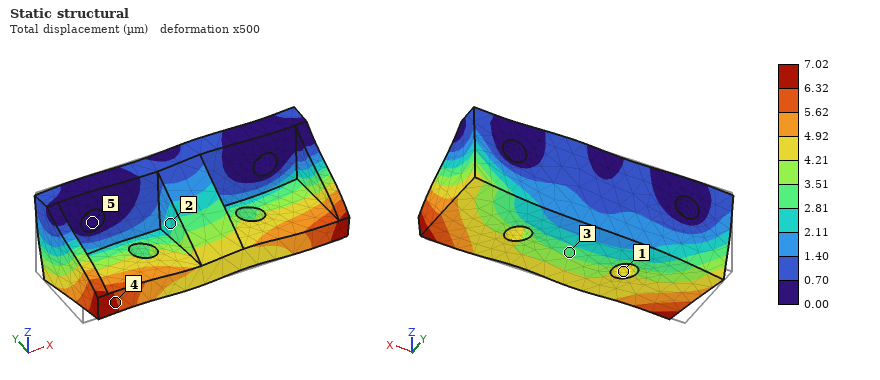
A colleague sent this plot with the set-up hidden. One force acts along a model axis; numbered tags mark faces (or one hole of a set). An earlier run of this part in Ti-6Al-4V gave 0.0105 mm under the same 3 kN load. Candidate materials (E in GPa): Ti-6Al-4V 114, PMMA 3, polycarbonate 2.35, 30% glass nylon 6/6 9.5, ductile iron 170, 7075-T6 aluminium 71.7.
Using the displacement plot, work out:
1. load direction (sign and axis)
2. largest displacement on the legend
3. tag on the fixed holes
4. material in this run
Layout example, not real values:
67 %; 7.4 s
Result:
+X; 7.02 µm; 5; ductile iron
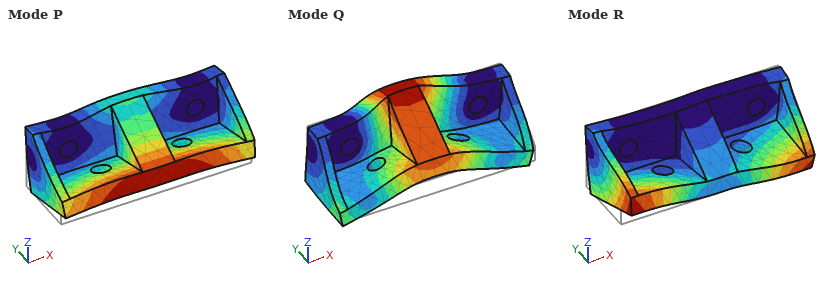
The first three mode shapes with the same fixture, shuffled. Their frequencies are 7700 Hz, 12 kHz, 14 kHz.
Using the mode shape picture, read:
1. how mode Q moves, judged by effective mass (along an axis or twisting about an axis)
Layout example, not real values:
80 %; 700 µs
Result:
along Y
